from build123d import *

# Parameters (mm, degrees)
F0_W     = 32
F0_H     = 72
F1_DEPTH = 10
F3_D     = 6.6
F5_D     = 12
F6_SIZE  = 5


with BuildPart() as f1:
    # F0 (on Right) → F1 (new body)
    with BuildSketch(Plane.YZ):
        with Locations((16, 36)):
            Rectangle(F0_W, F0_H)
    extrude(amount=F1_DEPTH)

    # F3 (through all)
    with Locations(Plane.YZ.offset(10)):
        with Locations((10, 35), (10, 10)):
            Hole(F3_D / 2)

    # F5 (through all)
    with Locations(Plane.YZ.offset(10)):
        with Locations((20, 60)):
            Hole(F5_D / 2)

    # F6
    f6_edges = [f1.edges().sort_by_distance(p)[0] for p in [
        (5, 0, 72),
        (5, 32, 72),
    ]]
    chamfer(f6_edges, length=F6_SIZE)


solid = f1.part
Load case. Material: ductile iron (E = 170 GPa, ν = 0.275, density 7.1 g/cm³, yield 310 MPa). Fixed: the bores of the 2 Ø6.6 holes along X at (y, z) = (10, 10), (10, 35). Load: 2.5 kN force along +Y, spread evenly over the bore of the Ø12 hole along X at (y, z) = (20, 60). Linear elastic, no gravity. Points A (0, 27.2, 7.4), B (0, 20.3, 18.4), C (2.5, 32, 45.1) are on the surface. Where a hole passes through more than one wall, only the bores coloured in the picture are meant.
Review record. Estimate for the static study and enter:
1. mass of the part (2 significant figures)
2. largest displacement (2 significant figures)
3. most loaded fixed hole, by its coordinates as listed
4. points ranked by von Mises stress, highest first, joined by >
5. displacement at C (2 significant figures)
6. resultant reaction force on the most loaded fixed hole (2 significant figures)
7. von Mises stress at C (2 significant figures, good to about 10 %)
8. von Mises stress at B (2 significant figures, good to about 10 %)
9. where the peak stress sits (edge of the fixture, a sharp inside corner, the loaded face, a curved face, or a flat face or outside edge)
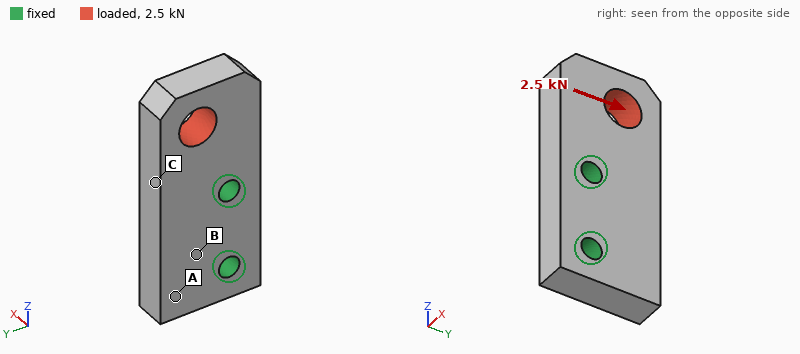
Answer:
150 g
18 µm
(10, 35)
C > B > A
7.2 µm
4.2 kN
27 MPa
15 MPa
edge of the fixture
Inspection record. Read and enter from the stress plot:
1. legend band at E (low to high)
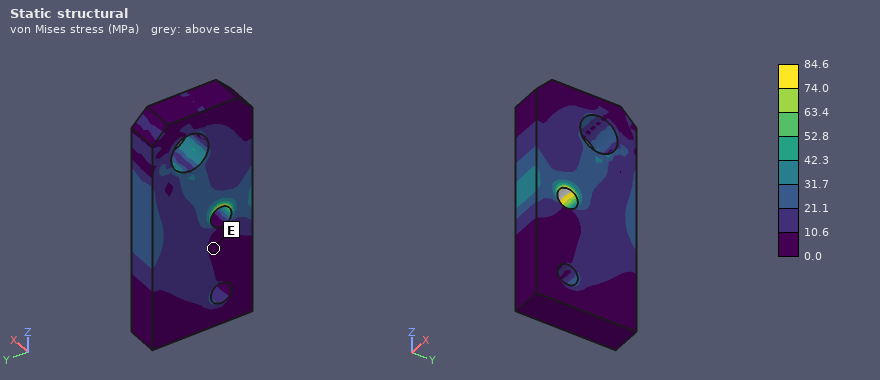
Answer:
0.0 to 10.6 MPa
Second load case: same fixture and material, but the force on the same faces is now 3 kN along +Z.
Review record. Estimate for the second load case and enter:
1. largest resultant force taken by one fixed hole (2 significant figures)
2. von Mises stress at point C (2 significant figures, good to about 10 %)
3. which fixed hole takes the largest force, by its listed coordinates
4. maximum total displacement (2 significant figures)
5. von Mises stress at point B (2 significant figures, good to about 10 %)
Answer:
2.3 kN
18 MPa
(10, 35)
6.8 µm
9.0 MPa
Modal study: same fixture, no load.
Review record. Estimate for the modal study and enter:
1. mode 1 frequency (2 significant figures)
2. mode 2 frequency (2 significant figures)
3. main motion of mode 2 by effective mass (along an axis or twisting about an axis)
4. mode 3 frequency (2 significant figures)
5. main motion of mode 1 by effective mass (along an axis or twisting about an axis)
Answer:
5600 Hz
9900 Hz
along Y
10 kHz
along X
